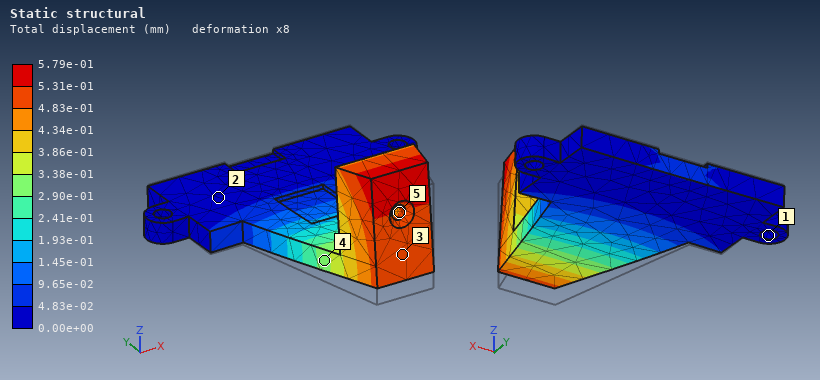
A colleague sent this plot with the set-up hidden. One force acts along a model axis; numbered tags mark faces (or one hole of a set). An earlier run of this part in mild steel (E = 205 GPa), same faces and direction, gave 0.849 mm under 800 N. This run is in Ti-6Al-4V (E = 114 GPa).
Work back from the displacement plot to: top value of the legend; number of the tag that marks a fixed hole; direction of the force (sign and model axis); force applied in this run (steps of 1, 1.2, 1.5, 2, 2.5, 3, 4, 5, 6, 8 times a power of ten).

5.79e-01 mm
1
+Z
300 N
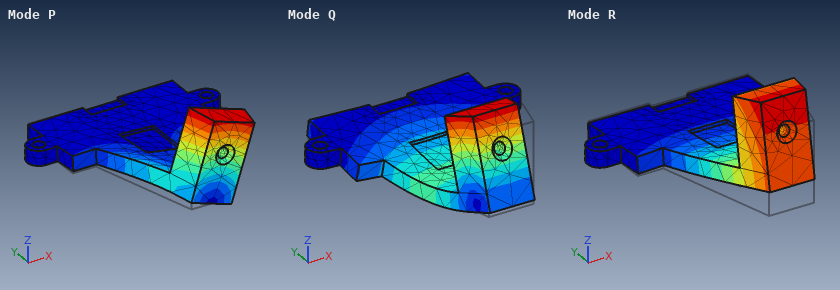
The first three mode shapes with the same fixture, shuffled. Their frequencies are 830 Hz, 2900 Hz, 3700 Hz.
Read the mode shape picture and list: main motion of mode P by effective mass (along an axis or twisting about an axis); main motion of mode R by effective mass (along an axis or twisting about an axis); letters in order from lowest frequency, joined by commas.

along X
along Z
R, P, Q
